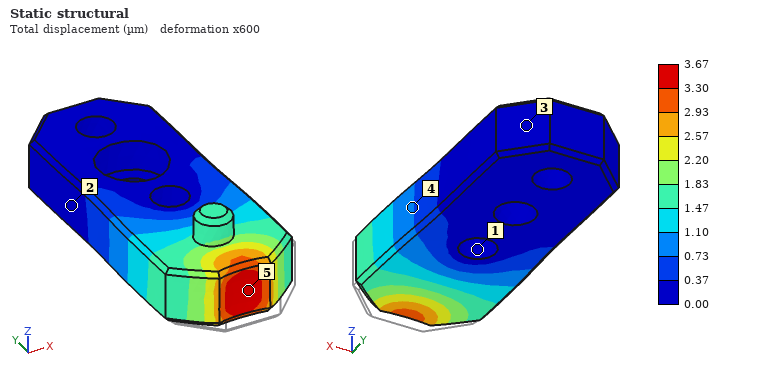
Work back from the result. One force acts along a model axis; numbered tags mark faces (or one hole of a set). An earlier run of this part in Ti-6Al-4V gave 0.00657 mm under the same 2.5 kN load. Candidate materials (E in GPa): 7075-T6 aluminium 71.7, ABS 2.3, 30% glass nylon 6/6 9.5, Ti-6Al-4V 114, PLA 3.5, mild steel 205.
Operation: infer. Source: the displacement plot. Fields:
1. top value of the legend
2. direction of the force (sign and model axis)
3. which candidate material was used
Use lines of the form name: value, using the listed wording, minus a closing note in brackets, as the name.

top value of the legend: 3.67 µm
direction of the force: +Y
which candidate material was used: mild steel
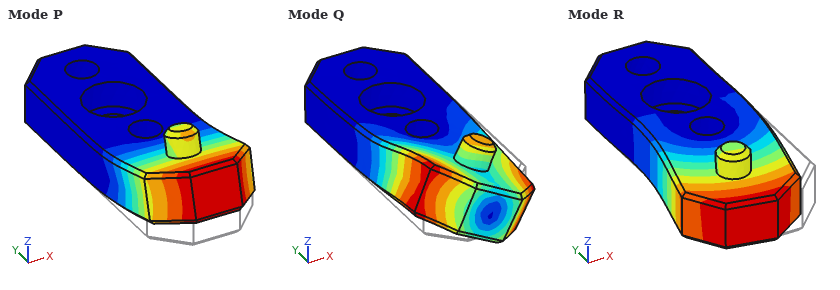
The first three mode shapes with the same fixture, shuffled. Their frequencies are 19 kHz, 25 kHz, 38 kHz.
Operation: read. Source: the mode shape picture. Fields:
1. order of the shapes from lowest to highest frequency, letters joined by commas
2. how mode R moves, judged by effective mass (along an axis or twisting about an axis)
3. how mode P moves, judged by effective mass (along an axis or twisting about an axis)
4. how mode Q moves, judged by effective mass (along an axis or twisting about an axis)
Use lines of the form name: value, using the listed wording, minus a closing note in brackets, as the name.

order of the shapes from lowest to highest frequency, letters joined by commas: P, R, Q
how mode R moves, judged by effective mass: along X
how mode P moves, judged by effective mass: along Z
how mode Q moves, judged by effective mass: twisting about Y
